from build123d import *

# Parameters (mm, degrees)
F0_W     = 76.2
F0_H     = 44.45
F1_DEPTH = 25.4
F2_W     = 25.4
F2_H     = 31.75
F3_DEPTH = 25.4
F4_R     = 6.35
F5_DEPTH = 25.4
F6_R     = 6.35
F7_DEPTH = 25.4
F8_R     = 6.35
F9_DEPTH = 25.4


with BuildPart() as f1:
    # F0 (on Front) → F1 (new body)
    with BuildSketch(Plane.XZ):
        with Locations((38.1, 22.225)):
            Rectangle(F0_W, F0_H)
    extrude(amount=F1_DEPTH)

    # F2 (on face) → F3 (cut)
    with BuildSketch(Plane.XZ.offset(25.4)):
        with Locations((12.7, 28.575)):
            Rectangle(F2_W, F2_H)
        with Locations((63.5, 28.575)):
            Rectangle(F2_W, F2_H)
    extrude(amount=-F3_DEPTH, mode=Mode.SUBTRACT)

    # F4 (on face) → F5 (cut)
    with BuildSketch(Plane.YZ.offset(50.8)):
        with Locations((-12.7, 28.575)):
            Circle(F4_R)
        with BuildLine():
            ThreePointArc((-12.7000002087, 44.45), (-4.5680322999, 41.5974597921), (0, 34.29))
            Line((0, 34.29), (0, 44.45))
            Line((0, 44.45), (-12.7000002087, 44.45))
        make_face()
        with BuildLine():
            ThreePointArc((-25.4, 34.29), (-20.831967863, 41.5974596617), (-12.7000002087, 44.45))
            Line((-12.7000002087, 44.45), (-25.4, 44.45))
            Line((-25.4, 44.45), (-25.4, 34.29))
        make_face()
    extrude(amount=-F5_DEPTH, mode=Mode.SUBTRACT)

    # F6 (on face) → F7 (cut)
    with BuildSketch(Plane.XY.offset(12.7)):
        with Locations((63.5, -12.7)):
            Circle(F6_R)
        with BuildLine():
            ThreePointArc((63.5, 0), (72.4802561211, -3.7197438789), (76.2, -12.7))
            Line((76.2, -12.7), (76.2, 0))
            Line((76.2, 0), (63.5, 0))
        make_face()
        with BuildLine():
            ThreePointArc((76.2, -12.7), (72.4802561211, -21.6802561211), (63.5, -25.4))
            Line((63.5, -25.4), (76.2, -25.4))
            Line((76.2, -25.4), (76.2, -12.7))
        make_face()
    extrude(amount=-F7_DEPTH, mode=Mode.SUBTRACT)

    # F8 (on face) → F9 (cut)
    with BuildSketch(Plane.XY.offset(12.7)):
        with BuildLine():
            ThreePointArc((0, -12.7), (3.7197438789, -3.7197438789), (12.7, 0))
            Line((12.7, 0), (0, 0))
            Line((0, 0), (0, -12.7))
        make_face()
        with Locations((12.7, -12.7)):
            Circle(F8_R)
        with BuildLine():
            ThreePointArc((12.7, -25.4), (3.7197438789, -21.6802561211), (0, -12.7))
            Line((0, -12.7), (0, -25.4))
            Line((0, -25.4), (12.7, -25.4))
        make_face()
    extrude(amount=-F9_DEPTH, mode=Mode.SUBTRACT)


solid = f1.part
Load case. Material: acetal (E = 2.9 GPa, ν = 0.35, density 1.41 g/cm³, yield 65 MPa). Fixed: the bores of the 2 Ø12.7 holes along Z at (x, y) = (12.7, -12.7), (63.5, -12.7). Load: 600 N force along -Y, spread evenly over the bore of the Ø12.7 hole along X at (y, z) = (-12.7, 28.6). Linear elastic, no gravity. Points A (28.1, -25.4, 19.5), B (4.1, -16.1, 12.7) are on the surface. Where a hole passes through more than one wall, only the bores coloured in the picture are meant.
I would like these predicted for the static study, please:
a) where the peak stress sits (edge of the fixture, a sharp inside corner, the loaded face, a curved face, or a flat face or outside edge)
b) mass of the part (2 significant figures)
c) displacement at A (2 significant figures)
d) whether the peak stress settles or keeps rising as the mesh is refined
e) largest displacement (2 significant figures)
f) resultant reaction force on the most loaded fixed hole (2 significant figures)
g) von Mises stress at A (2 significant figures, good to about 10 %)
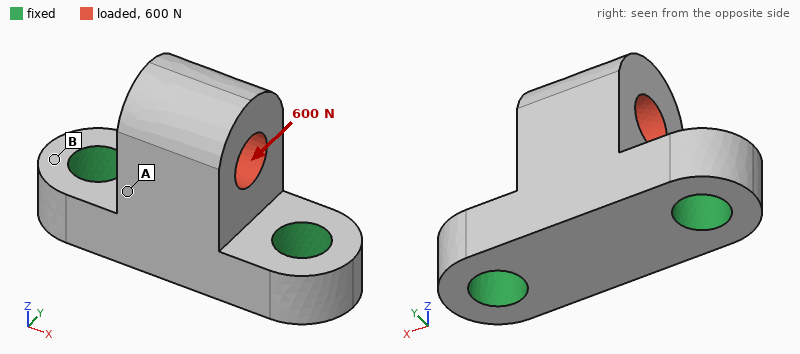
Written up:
edge of the fixture
50 g
0.12 mm
keeps rising
0.28 mm
300 N
3.8 MPa
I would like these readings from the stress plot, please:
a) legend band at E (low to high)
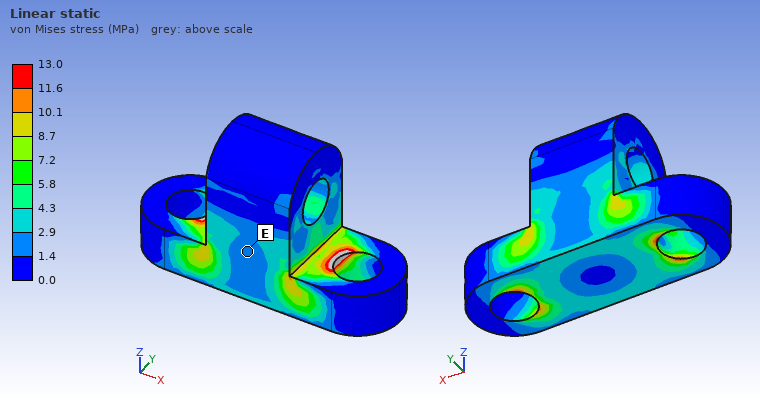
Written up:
1.4 to 2.9 MPa
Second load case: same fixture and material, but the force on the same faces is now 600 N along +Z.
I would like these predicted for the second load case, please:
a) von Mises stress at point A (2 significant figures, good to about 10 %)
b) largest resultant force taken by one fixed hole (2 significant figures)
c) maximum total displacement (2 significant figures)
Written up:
1.3 MPa
310 N
30 µm
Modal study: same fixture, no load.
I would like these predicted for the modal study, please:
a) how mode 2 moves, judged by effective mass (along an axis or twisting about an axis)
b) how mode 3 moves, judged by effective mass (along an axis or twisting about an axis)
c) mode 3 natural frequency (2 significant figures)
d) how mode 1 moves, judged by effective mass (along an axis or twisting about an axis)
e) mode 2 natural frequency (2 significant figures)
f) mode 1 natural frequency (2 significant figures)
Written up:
along X
along Z
4700 Hz
along Y
3200 Hz
1900 Hz
